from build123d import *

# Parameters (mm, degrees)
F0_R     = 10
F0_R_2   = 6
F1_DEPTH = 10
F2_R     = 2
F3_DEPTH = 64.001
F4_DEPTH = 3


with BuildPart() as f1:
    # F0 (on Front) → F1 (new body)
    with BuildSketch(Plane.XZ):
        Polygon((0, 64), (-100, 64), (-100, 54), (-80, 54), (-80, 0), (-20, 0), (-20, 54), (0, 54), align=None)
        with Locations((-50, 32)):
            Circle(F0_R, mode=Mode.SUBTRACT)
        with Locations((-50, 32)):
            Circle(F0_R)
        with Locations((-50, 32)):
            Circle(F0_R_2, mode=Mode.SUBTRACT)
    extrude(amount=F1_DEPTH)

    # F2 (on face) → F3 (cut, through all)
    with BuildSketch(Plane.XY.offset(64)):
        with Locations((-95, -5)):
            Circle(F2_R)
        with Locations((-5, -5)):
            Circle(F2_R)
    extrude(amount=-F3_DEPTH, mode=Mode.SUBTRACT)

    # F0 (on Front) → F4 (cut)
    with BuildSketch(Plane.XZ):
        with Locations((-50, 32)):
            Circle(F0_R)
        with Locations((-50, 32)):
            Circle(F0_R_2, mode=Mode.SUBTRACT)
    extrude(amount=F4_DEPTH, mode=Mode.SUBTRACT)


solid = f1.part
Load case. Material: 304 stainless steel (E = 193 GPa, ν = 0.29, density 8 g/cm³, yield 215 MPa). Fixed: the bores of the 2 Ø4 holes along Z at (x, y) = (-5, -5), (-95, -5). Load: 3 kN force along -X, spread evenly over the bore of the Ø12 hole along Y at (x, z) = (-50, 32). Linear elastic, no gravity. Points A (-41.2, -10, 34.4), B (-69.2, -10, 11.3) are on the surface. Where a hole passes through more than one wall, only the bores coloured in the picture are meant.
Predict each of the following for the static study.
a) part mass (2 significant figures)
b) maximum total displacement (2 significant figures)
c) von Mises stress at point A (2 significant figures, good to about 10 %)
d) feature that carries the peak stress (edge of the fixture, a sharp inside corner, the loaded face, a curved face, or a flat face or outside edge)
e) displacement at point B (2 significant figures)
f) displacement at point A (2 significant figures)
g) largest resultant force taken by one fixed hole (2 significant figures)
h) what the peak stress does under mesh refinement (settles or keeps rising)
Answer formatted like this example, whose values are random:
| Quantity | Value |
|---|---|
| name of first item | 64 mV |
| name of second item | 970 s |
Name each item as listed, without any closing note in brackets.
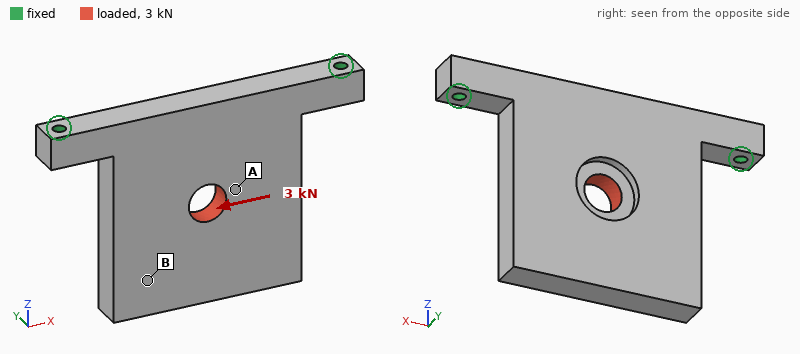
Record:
| Quantity | Value |
|---|---|
| part mass | 320 g |
| maximum total displacement | 17 µm |
| von Mises stress at point A | 15 MPa |
| feature that carries the peak stress | edge of the fixture |
| displacement at point B | 14 µm |
| displacement at point A | 8.1 µm |
| largest resultant force taken by one fixed hole | 1.9 kN |
| what the peak stress does under mesh refinement | keeps rising |
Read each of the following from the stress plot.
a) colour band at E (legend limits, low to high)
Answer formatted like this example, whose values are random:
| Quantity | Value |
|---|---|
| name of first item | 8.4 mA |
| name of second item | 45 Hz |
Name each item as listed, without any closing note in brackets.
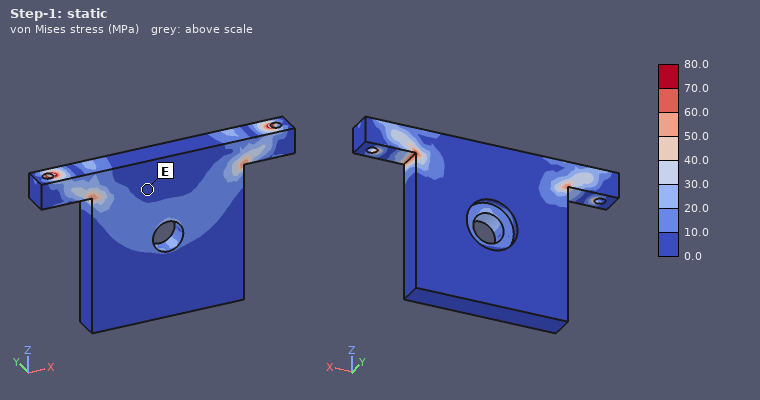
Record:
| Quantity | Value |
|---|---|
| colour band at E | 0.0 to 10.0 MPa |
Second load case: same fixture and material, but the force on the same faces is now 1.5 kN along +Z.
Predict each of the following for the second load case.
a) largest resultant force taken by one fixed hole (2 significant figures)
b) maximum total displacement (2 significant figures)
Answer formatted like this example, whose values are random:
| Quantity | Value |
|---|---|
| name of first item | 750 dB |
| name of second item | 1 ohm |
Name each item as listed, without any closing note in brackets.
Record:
| Quantity | Value |
|---|---|
| largest resultant force taken by one fixed hole | 860 N |
| maximum total displacement | 16 µm |
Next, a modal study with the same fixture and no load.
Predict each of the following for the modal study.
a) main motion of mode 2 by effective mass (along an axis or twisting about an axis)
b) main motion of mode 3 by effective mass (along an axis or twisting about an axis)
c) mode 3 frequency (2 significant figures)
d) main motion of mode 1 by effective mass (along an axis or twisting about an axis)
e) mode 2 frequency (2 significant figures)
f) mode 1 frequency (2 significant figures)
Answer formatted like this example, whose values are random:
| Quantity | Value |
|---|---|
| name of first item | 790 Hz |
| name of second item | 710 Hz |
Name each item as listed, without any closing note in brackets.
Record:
| Quantity | Value |
|---|---|
| main motion of mode 2 by effective mass | twisting about Z |
| main motion of mode 3 by effective mass | along X |
| mode 3 frequency | 4400 Hz |
| main motion of mode 1 by effective mass | along Y |
| mode 2 frequency | 3900 Hz |
| mode 1 frequency | 860 Hz |
